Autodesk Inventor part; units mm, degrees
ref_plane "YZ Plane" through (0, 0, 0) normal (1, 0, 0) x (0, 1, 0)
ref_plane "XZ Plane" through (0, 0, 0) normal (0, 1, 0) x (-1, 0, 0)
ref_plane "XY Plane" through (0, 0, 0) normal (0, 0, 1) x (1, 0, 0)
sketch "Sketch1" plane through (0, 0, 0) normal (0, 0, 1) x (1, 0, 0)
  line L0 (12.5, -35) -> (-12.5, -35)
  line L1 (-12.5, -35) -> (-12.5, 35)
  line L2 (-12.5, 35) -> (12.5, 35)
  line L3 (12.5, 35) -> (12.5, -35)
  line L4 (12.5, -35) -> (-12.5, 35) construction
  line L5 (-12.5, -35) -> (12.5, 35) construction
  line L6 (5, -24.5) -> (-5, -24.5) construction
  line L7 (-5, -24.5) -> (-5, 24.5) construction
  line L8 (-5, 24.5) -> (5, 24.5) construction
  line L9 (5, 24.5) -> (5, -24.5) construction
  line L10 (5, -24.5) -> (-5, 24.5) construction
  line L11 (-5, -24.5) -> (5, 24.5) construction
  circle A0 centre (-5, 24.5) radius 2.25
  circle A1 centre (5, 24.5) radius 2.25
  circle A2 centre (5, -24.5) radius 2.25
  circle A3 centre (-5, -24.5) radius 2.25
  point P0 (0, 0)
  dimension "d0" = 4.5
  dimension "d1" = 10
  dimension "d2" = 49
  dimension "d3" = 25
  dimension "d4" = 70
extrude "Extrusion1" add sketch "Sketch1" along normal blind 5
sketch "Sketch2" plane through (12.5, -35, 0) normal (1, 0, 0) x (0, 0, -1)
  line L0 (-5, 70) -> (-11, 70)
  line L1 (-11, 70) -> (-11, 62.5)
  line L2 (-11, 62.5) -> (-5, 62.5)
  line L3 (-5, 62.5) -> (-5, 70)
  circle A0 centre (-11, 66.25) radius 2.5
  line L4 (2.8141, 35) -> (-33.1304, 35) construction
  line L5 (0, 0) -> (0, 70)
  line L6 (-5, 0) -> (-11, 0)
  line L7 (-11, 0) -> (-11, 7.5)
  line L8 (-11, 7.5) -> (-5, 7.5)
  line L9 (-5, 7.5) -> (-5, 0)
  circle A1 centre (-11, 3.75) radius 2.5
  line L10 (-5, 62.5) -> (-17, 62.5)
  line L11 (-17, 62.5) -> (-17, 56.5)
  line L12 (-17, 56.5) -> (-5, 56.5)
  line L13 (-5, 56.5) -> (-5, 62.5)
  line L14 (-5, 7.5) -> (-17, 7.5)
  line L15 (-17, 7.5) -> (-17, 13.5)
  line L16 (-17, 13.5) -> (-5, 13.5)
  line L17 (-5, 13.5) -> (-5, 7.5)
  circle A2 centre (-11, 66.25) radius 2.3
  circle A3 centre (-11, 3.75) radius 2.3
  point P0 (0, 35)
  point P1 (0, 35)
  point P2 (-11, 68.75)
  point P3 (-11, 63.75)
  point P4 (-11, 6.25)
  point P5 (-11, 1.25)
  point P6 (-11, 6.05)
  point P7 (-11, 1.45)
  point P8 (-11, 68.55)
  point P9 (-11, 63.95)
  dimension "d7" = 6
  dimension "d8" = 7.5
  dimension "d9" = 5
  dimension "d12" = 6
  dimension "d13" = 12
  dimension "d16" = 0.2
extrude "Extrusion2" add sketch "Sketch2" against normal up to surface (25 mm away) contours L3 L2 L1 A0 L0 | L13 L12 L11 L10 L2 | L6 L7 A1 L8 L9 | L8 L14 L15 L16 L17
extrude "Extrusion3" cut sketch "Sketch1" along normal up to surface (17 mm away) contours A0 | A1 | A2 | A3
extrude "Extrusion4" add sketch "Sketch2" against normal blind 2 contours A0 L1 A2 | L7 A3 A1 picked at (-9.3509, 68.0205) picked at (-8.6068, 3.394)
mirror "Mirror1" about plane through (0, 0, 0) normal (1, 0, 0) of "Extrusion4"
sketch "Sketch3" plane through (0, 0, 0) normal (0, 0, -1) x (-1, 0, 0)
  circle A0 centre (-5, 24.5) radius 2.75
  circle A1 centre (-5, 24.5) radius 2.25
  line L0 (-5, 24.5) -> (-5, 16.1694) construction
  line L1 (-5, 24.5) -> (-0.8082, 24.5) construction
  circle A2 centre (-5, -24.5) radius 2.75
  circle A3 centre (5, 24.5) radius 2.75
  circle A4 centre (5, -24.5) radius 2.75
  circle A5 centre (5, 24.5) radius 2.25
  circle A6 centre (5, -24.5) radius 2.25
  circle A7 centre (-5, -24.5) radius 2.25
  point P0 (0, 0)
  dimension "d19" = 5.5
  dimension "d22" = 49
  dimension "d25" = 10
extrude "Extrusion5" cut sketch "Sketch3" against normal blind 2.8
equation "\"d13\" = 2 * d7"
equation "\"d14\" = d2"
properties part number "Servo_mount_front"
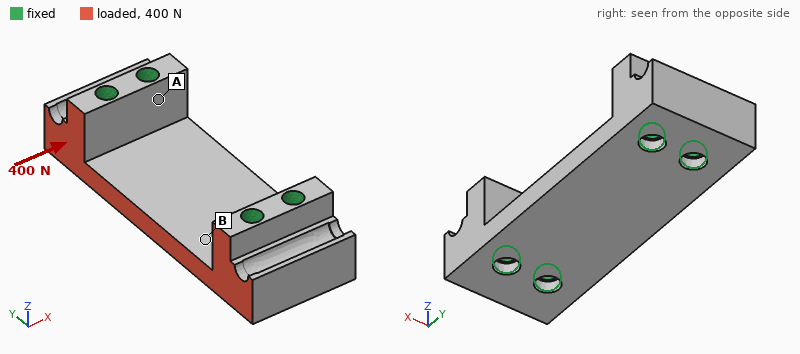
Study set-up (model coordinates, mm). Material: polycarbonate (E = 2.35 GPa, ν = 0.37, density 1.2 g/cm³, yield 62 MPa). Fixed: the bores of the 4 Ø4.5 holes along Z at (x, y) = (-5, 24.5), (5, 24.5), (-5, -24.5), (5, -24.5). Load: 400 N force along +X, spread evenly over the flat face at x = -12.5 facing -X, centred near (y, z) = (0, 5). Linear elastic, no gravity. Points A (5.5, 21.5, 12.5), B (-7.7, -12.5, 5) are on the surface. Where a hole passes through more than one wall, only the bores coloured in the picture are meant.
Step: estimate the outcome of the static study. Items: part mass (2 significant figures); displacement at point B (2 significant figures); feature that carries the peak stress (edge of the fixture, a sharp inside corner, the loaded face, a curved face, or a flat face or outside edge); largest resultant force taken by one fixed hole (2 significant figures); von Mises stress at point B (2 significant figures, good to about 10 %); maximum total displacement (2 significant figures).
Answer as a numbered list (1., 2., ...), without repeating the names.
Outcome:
1. 16 g
2. 12 µm
3. edge of the fixture
4. 140 N
5. 0.81 MPa
6. 18 µm
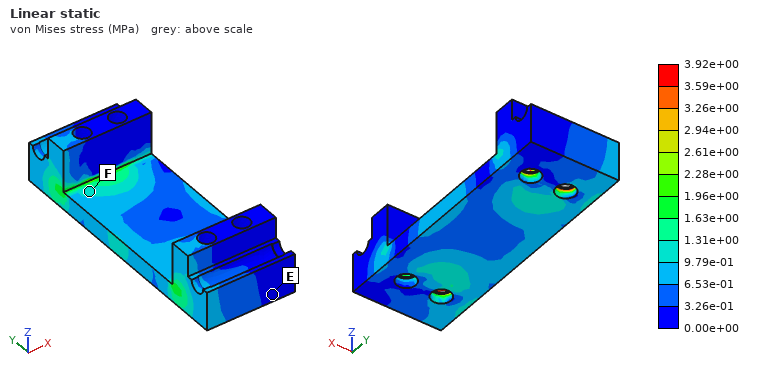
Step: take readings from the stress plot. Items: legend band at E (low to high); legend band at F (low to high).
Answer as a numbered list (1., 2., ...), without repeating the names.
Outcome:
1. 0.00e+00 to 3.26e-01 MPa
2. 9.79e-01 to 1.31e+00 MPa
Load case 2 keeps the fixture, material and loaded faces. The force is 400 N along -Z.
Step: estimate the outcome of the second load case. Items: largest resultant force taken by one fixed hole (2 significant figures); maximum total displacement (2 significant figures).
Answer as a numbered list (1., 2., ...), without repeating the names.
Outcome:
1. 240 N
2. 0.24 mm
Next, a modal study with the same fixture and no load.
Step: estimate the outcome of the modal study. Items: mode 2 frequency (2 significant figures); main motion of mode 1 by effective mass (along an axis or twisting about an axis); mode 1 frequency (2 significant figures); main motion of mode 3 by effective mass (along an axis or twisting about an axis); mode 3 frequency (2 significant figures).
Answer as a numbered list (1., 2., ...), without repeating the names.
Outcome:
1. 4300 Hz
2. along Z
3. 2900 Hz
4. along X
5. 6500 Hz
